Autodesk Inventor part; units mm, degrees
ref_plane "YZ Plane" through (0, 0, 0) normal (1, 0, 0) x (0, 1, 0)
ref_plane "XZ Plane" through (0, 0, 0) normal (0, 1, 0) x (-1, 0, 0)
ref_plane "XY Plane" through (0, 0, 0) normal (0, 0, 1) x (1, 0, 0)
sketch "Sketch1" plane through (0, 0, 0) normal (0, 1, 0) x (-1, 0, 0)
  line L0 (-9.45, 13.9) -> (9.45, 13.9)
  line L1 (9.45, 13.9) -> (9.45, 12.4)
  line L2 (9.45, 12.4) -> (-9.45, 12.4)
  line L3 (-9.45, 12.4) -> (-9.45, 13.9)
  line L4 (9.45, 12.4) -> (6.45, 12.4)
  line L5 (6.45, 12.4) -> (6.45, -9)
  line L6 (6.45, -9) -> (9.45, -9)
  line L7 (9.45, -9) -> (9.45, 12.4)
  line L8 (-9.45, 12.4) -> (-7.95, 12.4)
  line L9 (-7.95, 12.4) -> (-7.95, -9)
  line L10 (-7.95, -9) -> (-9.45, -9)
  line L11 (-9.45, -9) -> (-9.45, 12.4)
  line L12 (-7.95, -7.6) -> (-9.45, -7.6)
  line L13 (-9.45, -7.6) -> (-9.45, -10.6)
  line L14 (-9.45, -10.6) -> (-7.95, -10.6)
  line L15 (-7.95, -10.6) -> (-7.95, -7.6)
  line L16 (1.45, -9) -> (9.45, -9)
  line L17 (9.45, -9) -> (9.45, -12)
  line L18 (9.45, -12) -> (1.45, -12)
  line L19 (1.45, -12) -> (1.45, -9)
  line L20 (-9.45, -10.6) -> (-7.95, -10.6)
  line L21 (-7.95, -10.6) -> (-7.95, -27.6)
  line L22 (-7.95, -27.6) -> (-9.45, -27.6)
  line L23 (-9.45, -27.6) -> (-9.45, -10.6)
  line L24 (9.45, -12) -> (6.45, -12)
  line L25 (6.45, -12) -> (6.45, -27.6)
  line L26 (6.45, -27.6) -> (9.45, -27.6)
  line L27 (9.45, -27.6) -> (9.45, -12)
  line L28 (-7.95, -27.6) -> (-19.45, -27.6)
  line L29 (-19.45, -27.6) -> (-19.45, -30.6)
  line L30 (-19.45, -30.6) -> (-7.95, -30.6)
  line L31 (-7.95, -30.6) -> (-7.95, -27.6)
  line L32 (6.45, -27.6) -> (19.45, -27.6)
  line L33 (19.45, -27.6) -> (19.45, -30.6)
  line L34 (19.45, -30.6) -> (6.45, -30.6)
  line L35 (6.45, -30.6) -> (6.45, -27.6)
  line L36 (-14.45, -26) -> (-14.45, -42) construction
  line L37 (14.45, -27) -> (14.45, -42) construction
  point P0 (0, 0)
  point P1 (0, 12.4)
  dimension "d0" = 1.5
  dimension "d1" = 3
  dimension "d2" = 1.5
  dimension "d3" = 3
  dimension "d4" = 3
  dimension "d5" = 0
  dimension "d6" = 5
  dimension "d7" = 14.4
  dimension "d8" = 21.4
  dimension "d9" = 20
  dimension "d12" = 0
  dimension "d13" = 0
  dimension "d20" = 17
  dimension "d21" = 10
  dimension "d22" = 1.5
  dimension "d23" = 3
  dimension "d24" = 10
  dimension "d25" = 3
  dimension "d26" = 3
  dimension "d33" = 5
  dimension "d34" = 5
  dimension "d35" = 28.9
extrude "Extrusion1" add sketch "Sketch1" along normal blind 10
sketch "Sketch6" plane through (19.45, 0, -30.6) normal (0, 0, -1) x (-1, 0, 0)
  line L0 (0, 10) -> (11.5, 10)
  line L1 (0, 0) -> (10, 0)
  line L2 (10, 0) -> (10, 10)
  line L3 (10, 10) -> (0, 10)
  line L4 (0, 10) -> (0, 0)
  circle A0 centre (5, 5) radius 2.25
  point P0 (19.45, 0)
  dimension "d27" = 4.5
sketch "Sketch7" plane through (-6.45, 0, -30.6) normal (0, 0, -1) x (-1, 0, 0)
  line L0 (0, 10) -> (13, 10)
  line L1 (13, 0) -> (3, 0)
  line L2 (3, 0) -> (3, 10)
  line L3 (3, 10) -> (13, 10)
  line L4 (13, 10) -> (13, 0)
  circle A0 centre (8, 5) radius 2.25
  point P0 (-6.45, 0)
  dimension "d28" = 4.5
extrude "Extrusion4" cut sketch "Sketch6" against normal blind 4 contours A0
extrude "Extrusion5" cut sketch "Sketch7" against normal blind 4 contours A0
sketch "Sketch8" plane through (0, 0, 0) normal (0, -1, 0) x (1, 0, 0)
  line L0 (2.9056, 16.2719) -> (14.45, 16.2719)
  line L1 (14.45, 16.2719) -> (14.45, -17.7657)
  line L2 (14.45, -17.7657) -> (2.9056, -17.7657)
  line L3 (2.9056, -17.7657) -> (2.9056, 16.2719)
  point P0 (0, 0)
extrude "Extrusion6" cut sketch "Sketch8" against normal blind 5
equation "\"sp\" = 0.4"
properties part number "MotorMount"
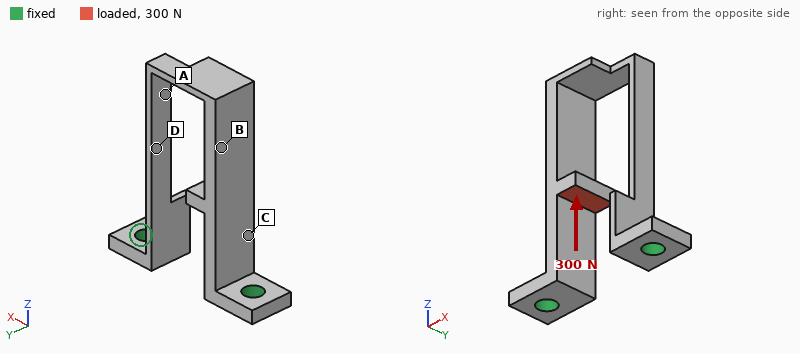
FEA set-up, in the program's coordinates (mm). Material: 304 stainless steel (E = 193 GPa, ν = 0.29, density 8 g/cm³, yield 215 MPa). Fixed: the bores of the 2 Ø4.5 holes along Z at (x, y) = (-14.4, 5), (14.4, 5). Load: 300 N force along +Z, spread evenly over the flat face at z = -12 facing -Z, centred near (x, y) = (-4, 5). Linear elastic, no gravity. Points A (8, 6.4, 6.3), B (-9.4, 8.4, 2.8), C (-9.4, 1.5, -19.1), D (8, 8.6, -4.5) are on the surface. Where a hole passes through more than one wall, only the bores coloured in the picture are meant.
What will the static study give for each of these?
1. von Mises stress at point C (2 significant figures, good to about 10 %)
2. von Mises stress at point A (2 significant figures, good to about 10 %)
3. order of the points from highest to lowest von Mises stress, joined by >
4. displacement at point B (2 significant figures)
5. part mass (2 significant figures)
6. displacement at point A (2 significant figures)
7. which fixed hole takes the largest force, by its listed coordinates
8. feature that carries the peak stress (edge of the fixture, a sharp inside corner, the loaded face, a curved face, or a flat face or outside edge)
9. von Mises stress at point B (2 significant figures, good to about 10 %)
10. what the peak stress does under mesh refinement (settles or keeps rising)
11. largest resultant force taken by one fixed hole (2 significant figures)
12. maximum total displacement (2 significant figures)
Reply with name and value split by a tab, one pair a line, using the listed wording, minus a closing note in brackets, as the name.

von Mises stress at point C	33 MPa
von Mises stress at point A	53 MPa
order of the points from highest to lowest von Mises stress, joined by >	A > C > B > D
displacement at point B	0.095 mm
part mass	21 g
displacement at point A	0.11 mm
which fixed hole takes the largest force, by its listed coordinates	(-14.4, 5)
feature that carries the peak stress	edge of the fixture
von Mises stress at point B	25 MPa
what the peak stress does under mesh refinement	keeps rising
largest resultant force taken by one fixed hole	270 N
maximum total displacement	0.12 mm
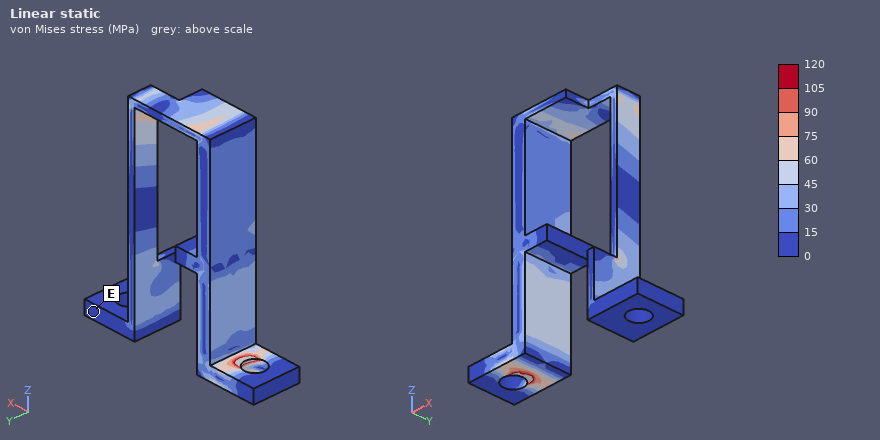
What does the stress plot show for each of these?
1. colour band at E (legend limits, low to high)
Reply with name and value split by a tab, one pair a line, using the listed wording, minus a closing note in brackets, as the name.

colour band at E	0 to 15 MPa
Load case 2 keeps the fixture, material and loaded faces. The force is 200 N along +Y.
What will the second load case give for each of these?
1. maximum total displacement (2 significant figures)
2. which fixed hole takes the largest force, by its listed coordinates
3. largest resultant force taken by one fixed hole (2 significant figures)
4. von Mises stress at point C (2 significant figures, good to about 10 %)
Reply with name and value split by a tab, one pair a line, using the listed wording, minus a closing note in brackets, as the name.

maximum total displacement	83 µm
which fixed hole takes the largest force, by its listed coordinates	(-14.4, 5)
largest resultant force taken by one fixed hole	180 N
von Mises stress at point C	23 MPa
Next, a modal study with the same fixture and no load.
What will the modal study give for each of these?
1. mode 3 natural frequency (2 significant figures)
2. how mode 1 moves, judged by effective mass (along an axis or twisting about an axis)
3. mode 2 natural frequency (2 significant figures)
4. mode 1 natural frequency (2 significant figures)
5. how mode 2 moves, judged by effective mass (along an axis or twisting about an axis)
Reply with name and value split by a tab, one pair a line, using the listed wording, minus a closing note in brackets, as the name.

mode 3 natural frequency	4000 Hz
how mode 1 moves, judged by effective mass	along X
mode 2 natural frequency	2000 Hz
mode 1 natural frequency	1200 Hz
how mode 2 moves, judged by effective mass	along Y
